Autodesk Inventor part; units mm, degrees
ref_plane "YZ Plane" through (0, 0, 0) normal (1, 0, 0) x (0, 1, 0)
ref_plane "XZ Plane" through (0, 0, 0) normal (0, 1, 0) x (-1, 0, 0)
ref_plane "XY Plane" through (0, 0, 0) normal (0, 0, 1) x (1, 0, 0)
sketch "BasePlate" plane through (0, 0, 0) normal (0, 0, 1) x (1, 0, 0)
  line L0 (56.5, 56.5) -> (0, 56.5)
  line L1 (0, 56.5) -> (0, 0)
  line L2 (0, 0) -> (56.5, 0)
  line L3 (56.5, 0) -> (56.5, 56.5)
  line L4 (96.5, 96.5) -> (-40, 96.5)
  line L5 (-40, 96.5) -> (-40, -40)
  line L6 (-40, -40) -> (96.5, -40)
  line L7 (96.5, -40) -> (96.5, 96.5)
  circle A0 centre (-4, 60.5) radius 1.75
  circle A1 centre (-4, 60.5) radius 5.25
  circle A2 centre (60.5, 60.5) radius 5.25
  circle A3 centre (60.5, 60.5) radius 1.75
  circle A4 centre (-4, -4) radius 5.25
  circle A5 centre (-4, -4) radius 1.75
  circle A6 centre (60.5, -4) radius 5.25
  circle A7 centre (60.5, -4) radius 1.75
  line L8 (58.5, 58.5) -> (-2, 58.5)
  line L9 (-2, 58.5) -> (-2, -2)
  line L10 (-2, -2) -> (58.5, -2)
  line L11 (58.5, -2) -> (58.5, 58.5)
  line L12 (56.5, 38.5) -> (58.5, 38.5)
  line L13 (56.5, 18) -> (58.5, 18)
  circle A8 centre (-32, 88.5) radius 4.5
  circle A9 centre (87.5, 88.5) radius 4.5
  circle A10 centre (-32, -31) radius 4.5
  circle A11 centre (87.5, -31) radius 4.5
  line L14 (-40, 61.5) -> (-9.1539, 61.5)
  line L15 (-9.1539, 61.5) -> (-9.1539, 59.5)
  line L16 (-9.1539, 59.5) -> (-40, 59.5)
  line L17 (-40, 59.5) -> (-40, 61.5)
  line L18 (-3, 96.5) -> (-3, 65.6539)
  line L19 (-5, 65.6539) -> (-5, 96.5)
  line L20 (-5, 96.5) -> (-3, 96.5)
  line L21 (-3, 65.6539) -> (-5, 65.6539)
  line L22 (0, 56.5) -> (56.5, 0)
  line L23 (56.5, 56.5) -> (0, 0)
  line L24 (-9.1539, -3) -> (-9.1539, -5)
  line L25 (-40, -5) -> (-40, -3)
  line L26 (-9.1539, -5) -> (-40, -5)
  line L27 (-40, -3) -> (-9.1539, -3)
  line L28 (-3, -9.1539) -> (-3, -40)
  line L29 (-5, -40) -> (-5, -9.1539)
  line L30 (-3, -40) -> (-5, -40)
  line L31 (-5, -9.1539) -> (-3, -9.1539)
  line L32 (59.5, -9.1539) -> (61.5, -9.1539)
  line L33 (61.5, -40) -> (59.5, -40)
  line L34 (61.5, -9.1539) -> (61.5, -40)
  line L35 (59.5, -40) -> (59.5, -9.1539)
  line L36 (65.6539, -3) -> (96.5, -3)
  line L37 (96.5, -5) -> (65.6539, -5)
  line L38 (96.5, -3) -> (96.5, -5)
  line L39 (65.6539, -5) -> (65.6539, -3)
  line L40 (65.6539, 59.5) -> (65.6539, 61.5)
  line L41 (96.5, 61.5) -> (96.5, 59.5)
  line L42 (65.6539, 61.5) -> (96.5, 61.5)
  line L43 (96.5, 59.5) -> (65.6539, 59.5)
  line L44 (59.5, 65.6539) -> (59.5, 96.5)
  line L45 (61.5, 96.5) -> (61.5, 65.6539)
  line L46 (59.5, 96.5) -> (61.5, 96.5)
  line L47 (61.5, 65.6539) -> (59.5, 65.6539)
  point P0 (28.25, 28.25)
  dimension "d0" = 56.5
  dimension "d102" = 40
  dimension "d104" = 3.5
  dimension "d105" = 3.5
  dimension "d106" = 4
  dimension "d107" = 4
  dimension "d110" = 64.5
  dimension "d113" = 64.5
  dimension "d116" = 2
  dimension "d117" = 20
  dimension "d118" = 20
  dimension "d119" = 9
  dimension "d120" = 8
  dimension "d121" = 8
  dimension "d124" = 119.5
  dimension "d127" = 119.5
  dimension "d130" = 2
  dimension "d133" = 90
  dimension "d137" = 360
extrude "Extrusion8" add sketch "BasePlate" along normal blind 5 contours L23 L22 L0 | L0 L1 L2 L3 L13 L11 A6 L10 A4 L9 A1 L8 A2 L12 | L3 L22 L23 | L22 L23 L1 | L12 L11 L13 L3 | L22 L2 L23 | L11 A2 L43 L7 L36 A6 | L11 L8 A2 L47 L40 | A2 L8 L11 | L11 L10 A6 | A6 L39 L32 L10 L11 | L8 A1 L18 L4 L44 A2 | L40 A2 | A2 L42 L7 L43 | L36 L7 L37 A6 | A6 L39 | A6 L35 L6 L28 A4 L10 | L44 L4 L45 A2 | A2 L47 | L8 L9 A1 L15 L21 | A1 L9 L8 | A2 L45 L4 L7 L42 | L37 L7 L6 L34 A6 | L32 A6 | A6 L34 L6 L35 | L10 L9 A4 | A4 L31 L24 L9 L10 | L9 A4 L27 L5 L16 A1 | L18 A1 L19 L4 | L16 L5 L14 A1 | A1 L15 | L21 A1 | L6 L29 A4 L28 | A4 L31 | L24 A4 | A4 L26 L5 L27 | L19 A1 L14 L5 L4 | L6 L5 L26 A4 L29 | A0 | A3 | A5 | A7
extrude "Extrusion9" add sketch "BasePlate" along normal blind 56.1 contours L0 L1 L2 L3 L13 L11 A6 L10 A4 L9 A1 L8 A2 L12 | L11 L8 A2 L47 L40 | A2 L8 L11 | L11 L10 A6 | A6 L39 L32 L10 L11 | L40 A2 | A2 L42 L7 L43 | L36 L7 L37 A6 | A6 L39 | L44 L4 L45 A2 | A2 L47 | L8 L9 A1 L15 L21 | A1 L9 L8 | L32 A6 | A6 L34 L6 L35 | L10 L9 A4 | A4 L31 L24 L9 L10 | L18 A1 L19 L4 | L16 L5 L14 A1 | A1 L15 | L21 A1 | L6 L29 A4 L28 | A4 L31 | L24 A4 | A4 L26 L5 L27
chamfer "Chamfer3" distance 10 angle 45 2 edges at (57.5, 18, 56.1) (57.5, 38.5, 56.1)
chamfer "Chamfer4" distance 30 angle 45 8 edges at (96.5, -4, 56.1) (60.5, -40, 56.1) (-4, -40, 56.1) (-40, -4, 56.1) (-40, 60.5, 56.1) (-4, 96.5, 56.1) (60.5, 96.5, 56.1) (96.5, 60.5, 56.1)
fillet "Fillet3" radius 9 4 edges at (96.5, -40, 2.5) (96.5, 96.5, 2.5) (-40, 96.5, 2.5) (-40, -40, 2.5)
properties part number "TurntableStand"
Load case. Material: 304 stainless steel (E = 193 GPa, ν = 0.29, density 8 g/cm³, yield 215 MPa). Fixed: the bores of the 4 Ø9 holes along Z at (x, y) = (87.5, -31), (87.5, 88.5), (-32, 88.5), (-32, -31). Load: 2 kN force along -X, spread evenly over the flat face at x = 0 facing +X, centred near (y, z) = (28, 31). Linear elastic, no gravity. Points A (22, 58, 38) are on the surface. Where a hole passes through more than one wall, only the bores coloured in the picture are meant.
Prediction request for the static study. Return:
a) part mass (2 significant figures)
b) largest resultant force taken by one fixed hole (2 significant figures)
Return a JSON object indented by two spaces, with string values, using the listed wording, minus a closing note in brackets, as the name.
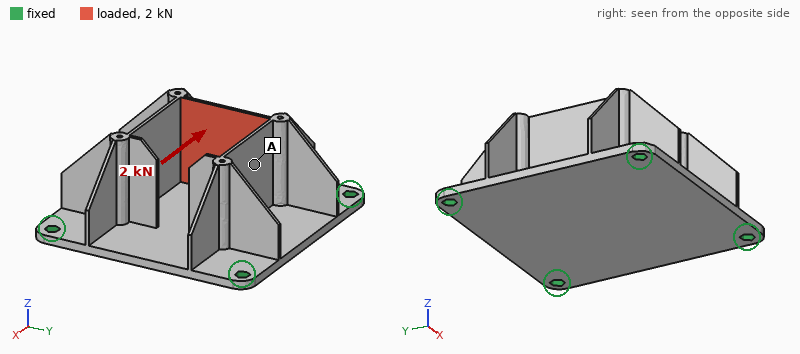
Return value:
{
  "part mass": "1.2 kg",
  "largest resultant force taken by one fixed hole": "640 N"
}
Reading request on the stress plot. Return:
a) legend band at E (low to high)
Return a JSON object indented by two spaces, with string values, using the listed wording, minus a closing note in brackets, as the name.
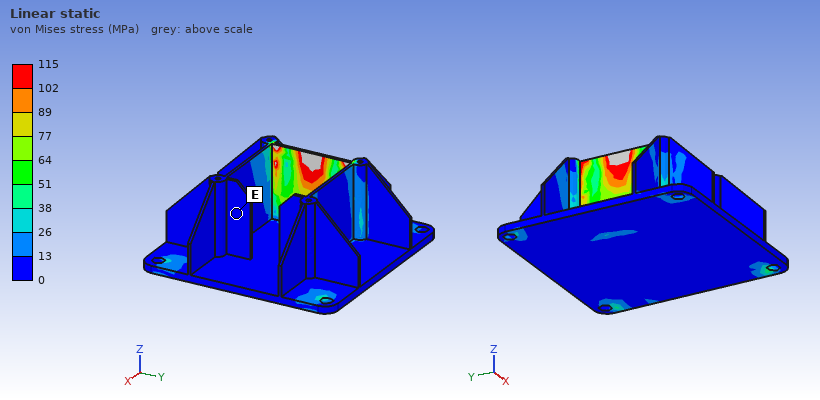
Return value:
{
  "legend band at E": "0 to 13 MPa"
}
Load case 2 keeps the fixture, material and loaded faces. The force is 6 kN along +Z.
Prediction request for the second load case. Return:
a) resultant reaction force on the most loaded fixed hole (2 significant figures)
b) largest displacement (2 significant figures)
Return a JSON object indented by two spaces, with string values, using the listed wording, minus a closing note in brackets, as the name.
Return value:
{
  "resultant reaction force on the most loaded fixed hole": "2.4 kN",
  "largest displacement": "0.10 mm"
}
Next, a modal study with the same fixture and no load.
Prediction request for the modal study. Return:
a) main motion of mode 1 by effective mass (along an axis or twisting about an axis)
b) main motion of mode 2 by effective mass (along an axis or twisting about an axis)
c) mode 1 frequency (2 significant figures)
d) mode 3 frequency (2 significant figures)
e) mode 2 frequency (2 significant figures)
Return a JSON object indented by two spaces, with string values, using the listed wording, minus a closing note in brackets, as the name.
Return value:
{
  "main motion of mode 1 by effective mass": "along Z",
  "main motion of mode 2 by effective mass": "along Z",
  "mode 1 frequency": "1400 Hz",
  "mode 3 frequency": "2200 Hz",
  "mode 2 frequency": "1900 Hz"
}
